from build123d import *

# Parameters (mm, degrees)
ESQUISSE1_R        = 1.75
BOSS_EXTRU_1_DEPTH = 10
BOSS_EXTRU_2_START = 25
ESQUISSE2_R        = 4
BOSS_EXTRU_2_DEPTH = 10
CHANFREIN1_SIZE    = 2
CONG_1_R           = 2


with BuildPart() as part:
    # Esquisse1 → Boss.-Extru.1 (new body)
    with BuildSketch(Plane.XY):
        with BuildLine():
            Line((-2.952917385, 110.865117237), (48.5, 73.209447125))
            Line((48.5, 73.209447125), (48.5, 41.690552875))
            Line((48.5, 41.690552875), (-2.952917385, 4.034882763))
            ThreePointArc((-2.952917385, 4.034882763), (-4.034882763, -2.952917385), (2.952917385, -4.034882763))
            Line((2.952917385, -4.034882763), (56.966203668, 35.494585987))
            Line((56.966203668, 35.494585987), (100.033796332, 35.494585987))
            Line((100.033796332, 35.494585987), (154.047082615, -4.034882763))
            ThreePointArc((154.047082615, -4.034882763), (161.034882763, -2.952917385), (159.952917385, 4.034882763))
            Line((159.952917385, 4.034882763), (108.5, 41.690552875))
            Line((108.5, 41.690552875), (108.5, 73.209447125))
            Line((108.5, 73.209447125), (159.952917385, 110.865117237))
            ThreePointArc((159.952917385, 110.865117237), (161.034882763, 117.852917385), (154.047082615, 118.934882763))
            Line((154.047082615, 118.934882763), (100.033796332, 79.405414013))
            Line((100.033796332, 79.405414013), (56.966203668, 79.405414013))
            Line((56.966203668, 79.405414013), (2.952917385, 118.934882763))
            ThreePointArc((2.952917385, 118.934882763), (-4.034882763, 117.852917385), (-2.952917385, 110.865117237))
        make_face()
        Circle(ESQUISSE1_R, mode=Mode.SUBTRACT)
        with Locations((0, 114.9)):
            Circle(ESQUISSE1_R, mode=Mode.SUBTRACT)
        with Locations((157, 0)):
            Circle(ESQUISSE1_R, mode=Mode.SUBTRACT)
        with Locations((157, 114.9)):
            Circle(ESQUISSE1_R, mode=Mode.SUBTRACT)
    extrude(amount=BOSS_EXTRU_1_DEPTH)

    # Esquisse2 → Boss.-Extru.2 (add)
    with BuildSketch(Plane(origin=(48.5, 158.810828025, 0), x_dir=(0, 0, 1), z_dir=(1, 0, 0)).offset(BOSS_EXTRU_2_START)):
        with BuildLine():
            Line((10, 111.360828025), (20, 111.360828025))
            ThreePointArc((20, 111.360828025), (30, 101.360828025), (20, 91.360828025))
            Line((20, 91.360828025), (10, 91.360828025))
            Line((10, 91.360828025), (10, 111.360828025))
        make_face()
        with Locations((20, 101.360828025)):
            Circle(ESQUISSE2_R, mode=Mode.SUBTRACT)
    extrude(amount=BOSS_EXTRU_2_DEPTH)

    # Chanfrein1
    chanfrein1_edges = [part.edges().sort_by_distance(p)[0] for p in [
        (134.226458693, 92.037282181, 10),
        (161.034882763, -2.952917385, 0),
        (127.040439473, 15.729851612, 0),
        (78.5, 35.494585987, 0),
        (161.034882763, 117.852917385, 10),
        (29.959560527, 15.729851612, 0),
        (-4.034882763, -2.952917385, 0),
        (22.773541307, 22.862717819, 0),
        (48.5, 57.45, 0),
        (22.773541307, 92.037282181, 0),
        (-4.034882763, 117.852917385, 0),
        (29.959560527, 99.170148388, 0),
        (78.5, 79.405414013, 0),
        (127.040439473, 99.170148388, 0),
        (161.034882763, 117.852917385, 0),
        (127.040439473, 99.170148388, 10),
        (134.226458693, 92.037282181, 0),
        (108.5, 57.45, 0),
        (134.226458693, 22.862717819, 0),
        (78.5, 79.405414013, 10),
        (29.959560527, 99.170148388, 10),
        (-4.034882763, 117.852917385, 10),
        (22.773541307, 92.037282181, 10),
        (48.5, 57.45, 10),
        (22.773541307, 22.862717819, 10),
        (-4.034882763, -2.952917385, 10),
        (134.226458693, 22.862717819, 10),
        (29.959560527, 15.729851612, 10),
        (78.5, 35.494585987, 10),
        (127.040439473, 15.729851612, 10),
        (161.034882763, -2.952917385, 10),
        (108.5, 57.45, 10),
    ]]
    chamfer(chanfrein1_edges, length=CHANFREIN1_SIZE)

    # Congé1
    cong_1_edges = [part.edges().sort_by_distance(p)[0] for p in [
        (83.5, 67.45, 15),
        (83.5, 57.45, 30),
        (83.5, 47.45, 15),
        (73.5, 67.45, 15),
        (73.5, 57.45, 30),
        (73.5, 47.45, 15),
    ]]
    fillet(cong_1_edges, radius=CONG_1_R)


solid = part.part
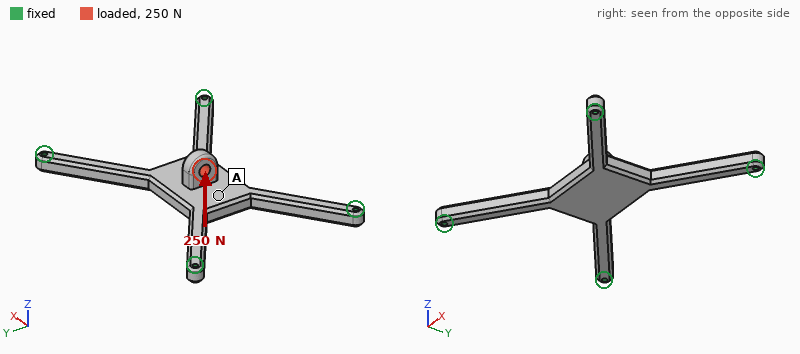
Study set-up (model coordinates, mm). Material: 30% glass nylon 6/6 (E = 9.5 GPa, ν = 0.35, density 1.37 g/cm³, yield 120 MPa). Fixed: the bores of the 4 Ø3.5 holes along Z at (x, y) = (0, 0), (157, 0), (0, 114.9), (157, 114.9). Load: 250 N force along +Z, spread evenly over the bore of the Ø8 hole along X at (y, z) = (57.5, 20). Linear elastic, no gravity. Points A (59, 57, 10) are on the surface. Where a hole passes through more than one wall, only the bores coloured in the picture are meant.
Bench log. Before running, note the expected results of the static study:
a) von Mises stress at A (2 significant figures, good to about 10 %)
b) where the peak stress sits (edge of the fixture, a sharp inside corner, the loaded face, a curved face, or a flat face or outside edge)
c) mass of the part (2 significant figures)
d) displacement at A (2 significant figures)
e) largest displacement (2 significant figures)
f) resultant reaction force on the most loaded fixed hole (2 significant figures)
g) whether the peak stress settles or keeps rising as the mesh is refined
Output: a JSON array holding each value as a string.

["3.7 MPa", "edge of the fixture", "72 g", "0.38 mm", "0.40 mm", "63 N", "keeps rising"]
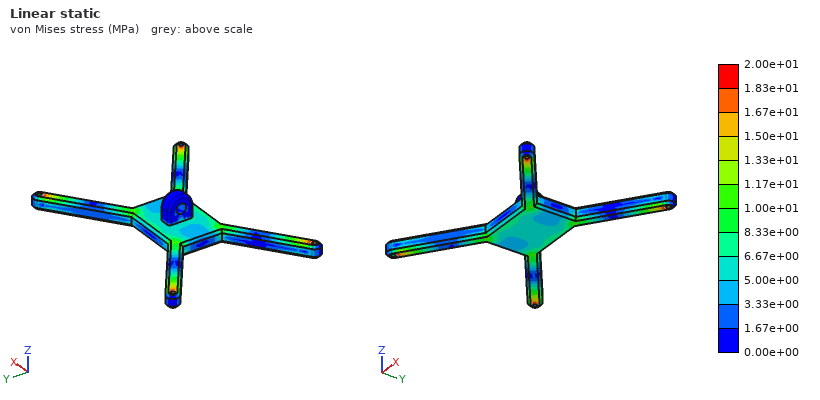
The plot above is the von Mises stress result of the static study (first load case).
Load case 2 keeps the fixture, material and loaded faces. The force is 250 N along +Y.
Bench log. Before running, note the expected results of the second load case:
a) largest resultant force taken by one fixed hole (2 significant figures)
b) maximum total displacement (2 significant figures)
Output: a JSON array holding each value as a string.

["100 N", "0.12 mm"]
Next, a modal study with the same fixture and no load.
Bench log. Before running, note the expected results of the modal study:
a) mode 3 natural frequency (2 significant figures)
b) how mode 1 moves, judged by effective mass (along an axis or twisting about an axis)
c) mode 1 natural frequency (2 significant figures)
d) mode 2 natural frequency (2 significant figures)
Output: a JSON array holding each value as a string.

["1600 Hz", "along Z", "600 Hz", "1600 Hz"]
